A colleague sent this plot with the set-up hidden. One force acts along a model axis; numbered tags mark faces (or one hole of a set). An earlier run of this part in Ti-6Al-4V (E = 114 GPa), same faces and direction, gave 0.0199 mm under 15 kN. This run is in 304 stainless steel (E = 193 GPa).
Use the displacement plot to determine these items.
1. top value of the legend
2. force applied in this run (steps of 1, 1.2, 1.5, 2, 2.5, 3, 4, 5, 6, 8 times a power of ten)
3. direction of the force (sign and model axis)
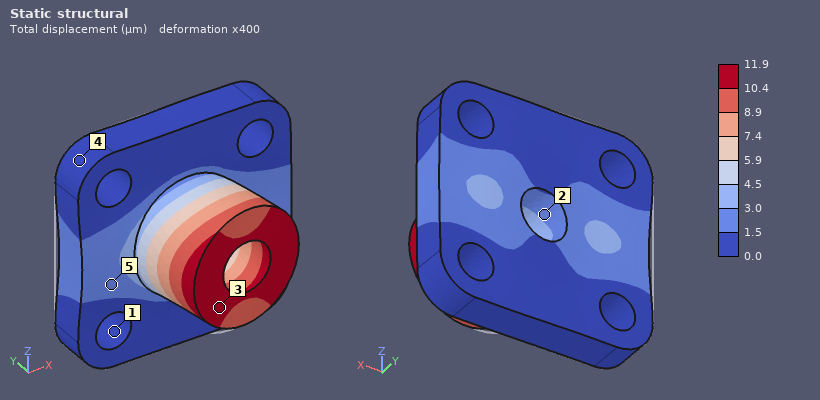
11.9 µm
15 kN
+X
